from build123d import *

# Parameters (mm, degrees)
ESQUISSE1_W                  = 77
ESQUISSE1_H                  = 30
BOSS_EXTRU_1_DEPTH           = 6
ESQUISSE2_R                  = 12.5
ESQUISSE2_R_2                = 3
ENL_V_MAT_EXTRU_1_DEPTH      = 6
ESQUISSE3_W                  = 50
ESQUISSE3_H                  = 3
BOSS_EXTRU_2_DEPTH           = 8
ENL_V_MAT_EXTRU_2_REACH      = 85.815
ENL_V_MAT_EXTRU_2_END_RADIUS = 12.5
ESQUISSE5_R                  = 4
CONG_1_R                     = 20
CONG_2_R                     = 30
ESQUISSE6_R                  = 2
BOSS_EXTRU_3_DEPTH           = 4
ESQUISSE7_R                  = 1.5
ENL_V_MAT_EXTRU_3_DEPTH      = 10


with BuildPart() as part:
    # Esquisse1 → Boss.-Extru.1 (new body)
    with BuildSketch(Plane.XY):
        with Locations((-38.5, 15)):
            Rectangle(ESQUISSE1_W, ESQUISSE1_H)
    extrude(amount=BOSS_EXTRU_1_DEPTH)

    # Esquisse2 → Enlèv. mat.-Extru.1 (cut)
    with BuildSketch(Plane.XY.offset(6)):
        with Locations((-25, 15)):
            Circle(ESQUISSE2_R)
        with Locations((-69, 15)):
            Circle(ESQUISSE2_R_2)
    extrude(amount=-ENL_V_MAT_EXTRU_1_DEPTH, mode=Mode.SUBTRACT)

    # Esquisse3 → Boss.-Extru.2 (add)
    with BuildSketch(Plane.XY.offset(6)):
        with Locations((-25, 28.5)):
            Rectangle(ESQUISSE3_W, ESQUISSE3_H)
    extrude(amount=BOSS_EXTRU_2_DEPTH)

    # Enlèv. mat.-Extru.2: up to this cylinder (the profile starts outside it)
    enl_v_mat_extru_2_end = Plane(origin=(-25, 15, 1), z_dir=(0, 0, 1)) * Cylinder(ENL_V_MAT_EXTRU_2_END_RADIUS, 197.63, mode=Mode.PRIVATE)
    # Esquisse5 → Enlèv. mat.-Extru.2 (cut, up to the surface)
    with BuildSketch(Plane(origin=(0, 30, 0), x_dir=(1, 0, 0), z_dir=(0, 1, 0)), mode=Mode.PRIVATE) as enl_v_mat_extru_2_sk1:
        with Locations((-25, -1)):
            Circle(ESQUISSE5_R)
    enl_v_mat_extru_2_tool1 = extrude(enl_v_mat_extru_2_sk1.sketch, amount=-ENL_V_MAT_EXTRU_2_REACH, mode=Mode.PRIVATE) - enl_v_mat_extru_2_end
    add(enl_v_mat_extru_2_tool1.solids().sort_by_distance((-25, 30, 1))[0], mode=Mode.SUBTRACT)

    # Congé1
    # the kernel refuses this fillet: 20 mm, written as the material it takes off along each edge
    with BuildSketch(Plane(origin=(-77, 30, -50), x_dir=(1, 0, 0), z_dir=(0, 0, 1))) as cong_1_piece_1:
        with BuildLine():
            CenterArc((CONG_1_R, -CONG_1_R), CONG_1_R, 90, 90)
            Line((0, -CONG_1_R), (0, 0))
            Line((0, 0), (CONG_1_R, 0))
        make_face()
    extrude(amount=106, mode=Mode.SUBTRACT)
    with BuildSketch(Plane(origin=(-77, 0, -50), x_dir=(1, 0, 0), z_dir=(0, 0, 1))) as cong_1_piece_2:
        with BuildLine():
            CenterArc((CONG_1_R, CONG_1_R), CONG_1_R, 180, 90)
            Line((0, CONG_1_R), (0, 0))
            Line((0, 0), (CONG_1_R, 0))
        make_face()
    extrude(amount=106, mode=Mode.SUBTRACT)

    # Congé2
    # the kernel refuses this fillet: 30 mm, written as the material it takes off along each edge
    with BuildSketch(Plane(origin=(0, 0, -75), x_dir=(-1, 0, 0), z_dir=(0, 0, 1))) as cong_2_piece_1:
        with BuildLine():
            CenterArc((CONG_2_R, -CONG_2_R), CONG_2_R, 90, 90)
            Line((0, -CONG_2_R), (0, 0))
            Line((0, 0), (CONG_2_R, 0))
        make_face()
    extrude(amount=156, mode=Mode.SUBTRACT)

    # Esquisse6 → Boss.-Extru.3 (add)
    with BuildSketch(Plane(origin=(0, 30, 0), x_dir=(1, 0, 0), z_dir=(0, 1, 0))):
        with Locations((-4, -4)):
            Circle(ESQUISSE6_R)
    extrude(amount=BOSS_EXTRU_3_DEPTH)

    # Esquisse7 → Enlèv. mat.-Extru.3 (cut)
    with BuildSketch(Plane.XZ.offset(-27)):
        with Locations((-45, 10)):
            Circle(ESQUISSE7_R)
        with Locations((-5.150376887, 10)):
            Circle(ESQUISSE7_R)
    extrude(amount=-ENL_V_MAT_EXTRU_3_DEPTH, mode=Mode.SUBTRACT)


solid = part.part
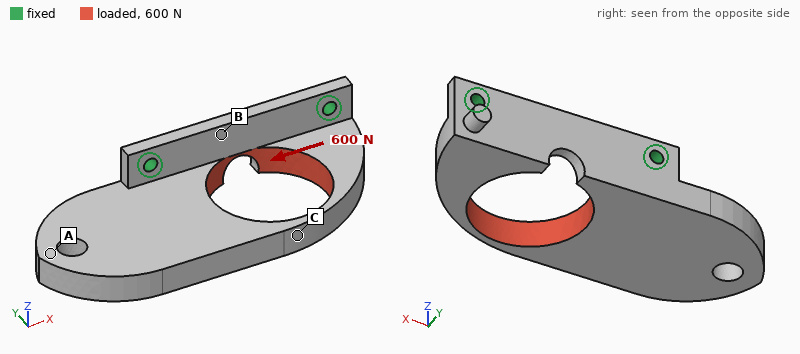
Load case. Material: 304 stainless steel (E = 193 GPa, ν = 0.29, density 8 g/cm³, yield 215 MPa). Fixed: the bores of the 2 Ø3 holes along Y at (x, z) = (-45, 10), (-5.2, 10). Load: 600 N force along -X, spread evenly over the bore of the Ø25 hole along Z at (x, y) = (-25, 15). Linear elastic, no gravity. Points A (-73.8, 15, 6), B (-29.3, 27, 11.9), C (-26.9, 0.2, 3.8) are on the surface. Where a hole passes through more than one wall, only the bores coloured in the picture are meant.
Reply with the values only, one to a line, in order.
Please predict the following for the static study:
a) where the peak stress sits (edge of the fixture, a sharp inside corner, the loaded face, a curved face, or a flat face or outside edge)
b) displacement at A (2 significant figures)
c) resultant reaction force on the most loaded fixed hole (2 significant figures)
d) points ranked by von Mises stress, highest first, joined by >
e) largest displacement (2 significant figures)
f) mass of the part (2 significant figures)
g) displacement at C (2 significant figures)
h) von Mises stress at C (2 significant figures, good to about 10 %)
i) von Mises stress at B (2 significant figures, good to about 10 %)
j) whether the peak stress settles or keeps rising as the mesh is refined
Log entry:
edge of the fixture
16 µm
360 N
C > B > A
18 µm
77 g
12 µm
37 MPa
14 MPa
keeps rising
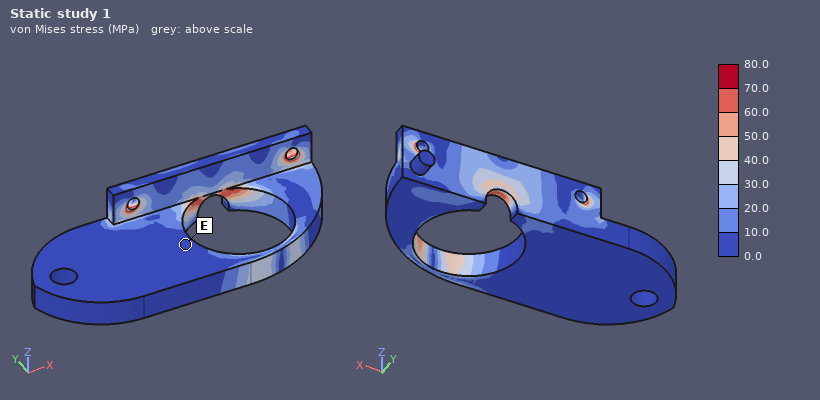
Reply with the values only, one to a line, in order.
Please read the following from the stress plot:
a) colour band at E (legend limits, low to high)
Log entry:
0.0 to 10.0 MPa
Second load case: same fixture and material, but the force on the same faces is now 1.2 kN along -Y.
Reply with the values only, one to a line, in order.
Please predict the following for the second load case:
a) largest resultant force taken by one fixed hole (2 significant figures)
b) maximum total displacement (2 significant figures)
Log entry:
620 N
67 µm
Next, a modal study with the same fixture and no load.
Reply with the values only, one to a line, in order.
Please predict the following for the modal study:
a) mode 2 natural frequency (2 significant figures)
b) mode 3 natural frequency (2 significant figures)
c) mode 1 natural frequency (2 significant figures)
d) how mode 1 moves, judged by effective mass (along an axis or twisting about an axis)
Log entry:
3800 Hz
4100 Hz
1600 Hz
along Z
